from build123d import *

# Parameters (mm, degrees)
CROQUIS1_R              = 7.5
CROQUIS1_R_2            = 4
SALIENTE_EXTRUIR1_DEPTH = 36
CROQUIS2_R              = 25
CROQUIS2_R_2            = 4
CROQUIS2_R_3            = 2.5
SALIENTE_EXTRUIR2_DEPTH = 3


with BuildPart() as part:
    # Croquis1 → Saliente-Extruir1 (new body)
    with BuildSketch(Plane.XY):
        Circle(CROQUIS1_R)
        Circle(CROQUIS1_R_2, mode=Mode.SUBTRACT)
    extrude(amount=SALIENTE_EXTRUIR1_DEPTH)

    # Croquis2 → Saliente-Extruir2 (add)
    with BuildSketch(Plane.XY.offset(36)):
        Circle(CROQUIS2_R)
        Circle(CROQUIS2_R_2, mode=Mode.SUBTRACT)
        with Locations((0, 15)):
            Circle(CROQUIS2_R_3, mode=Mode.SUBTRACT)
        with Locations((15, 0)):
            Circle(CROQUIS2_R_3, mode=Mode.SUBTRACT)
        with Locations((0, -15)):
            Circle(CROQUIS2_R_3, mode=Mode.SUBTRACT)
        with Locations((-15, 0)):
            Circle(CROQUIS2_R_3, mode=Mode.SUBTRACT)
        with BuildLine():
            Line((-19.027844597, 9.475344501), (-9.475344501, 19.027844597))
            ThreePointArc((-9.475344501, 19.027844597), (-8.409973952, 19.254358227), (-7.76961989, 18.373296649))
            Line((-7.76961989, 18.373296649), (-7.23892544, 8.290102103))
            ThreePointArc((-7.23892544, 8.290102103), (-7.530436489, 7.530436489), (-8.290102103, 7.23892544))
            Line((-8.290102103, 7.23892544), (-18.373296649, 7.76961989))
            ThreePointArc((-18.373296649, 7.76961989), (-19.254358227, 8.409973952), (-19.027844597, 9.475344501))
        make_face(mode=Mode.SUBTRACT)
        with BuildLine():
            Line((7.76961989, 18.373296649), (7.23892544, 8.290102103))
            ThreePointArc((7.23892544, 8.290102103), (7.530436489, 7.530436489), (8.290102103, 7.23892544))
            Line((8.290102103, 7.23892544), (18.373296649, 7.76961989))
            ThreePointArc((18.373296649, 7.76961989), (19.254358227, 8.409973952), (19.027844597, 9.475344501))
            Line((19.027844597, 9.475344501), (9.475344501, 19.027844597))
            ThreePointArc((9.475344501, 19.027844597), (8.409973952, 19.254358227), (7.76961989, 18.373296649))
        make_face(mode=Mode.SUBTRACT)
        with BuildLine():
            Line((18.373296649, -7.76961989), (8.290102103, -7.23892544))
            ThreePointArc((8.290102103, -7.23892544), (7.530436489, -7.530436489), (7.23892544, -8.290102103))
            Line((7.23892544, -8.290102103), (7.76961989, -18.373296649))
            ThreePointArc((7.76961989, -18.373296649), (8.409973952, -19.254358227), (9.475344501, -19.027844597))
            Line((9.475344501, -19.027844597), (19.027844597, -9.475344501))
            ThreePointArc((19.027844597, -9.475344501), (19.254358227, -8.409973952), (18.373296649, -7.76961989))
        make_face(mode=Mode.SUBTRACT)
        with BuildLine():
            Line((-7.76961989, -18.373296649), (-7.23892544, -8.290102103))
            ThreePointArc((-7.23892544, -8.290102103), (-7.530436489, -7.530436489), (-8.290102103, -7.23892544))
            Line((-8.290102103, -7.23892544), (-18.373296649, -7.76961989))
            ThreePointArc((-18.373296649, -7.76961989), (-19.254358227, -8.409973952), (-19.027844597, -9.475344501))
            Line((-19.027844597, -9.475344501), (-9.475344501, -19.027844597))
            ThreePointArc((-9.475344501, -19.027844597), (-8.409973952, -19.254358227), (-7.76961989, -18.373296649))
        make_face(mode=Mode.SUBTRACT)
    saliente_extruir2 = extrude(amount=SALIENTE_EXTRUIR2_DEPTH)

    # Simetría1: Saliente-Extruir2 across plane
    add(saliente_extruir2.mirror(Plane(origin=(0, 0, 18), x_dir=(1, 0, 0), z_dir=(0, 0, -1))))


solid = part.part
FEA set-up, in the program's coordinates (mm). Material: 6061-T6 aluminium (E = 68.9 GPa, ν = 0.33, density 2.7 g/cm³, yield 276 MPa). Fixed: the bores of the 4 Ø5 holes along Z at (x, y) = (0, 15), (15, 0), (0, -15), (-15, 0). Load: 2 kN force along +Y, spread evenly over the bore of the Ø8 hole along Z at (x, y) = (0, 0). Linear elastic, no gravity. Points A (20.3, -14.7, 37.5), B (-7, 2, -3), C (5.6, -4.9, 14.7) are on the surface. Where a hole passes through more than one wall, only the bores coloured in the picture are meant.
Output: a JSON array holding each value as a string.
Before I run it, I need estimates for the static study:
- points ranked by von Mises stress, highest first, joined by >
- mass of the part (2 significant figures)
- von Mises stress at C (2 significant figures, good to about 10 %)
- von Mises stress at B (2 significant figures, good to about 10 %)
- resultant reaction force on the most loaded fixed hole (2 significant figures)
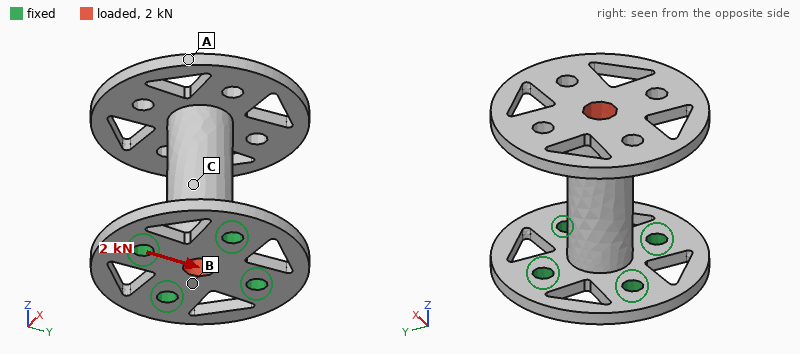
["B > C > A", "36 g", "35 MPa", "72 MPa", "1.9 kN"]
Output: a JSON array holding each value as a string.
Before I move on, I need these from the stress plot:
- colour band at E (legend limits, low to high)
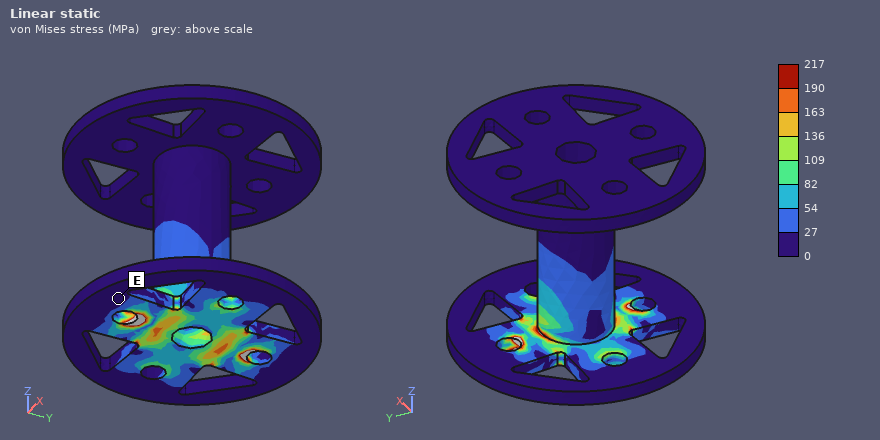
["0 to 27 MPa"]
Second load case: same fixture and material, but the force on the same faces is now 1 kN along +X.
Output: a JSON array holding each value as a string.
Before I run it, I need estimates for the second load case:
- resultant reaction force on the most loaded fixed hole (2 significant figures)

["940 N"]
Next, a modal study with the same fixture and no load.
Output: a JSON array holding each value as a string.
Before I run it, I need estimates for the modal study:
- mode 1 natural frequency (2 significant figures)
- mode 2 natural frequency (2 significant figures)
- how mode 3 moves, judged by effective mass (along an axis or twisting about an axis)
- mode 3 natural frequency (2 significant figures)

["2100 Hz", "2100 Hz", "twisting about Z", "4100 Hz"]
